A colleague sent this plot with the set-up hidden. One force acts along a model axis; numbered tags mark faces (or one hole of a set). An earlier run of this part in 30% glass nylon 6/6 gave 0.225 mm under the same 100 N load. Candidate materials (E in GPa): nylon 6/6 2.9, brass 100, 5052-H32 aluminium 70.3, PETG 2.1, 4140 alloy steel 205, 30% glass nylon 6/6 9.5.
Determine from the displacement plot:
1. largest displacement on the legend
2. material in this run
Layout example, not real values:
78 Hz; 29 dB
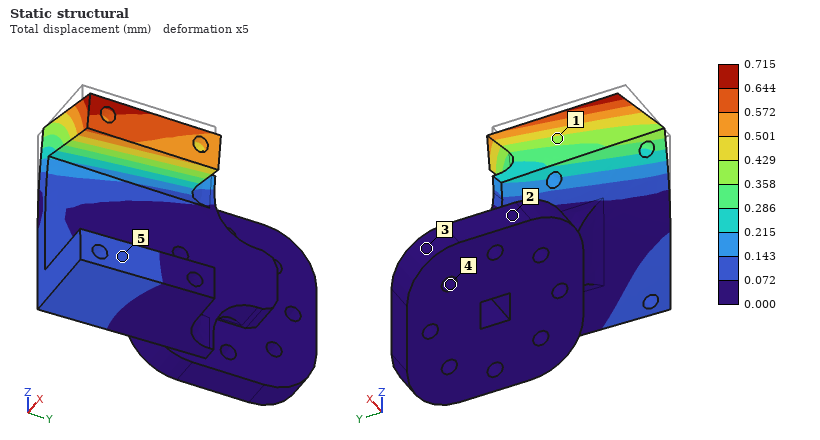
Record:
0.715 mm; nylon 6/6
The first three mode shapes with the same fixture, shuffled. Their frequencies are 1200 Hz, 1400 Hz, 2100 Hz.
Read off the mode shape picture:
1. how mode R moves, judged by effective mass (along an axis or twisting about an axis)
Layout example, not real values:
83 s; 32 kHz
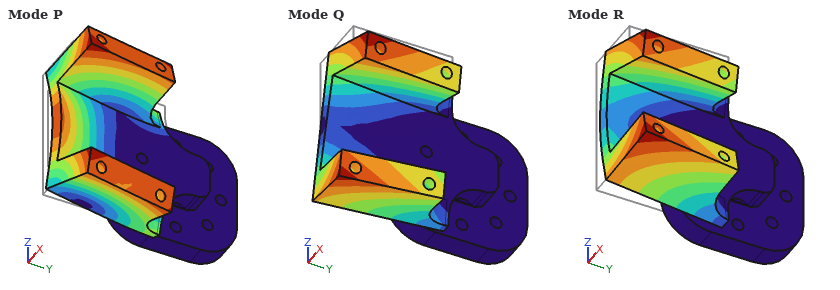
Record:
along X
